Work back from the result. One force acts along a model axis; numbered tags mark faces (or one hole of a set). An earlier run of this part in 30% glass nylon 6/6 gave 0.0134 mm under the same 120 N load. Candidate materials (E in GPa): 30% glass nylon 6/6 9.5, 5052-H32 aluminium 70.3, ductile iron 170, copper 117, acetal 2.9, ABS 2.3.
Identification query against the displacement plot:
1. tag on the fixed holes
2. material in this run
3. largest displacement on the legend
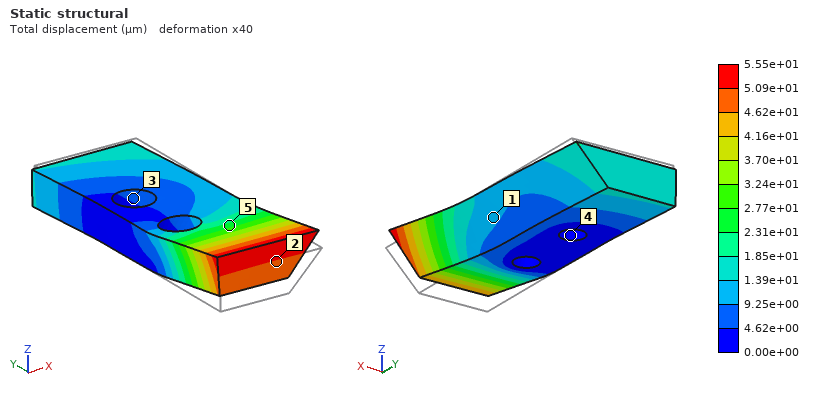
4
ABS
5.55e+01 µm
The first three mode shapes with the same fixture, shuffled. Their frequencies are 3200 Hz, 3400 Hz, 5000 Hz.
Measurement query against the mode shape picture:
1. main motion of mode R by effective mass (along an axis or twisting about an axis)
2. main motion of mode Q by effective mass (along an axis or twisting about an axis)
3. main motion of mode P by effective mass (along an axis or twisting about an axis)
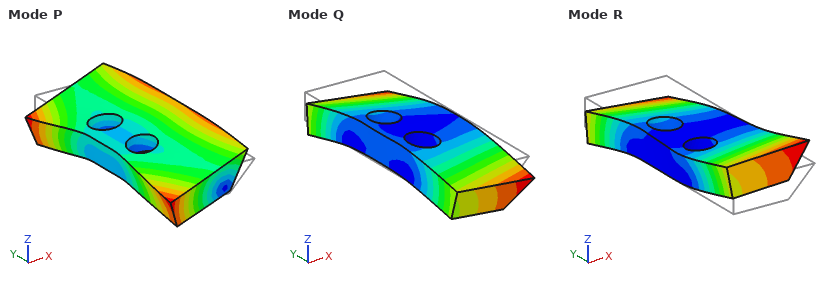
twisting about X
along Z
along X
